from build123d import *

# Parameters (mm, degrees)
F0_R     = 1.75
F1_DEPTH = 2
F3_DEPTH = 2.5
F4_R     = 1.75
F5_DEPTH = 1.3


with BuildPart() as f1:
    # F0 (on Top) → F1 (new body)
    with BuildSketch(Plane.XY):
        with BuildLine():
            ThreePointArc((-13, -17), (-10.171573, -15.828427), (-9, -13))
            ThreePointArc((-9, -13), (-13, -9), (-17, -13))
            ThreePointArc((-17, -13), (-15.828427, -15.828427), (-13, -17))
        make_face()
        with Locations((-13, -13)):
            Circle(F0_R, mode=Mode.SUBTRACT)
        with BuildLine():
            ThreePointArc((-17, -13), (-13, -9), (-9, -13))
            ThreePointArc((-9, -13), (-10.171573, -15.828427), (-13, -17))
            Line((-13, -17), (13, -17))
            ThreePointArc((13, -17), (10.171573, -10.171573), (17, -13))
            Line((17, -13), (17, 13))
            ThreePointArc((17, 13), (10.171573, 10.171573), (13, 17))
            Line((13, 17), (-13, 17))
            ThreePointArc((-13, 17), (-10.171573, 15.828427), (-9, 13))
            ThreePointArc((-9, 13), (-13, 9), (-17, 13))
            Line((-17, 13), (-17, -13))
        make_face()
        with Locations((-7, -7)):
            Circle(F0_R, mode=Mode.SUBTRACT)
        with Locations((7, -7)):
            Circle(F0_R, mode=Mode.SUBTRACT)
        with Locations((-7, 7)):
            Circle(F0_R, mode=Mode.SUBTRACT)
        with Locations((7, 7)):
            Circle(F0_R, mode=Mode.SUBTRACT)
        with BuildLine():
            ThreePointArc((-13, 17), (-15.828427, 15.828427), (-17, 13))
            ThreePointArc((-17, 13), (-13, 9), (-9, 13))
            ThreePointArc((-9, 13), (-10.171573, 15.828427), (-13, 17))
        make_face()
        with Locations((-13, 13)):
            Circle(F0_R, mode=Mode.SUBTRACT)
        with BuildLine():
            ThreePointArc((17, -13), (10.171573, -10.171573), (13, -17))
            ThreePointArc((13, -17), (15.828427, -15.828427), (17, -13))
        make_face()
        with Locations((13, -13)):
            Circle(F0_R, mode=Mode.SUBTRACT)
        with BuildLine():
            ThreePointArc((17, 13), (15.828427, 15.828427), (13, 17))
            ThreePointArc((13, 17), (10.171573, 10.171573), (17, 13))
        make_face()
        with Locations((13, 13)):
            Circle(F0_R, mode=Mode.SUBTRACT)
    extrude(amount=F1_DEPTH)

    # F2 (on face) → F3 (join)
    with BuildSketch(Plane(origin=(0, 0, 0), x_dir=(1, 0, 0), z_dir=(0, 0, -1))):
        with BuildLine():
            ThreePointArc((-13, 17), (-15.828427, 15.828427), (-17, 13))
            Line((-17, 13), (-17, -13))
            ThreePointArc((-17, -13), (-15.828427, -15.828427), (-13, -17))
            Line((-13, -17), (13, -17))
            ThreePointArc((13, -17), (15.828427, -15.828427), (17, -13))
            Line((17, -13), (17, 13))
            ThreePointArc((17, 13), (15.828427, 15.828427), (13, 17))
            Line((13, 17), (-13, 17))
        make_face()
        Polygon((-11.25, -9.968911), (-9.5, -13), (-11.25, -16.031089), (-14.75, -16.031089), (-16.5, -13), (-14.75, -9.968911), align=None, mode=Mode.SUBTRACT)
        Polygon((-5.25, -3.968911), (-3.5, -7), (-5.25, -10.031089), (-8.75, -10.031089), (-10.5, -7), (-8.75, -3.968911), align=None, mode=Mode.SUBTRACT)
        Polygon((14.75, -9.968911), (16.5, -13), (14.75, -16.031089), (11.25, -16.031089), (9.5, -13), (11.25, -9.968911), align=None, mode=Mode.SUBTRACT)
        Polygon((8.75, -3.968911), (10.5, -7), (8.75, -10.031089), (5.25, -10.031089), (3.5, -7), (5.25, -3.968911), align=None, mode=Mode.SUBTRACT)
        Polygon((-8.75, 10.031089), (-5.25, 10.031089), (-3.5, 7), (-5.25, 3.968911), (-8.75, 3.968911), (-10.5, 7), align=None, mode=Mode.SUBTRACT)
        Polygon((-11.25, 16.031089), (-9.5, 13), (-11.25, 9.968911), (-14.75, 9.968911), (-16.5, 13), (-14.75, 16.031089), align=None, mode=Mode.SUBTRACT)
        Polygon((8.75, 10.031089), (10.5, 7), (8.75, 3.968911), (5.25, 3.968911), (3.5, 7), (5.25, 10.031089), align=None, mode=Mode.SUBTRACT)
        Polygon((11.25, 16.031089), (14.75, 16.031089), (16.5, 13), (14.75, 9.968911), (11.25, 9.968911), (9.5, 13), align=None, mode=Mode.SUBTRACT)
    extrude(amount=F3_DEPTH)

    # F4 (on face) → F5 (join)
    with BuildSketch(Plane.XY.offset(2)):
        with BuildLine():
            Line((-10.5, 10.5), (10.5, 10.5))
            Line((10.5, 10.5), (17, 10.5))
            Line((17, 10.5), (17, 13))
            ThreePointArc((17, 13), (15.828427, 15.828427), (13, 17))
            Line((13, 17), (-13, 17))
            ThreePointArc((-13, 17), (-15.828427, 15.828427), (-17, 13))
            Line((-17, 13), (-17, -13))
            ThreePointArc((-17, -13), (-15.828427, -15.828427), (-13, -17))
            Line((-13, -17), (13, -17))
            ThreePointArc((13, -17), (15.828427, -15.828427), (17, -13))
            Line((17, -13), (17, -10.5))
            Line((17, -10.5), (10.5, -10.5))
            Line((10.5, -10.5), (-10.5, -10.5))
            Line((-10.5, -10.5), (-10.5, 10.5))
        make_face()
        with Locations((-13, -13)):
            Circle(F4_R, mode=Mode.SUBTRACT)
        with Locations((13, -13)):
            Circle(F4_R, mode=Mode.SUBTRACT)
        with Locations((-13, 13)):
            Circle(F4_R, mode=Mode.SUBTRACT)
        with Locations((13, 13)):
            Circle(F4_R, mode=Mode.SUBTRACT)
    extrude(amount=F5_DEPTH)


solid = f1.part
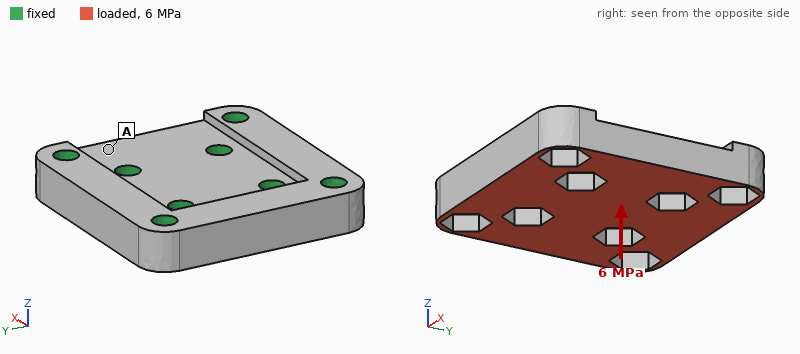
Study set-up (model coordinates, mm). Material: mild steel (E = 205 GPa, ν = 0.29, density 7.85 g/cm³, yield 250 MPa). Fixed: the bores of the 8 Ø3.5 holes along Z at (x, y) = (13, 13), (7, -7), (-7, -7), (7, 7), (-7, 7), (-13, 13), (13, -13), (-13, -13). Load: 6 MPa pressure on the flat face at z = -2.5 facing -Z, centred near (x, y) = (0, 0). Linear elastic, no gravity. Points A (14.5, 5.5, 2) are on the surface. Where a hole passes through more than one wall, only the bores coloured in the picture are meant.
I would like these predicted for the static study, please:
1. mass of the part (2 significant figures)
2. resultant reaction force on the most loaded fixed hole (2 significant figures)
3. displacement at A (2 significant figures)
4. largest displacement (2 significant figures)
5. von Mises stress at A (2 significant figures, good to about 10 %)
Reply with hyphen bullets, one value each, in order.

- 40 g
- 780 N
- 2.4 µm
- 4.3 µm
- 12 MPa
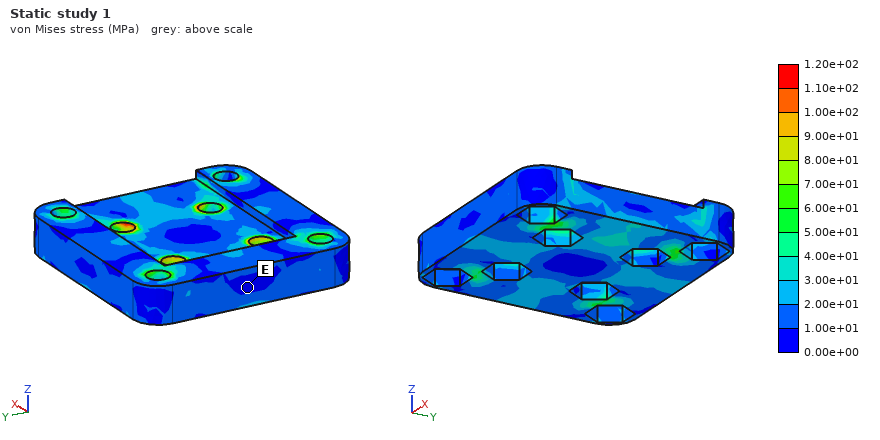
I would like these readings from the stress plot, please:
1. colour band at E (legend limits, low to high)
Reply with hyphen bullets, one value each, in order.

- 0.00e+00 to 1.00e+01 MPa
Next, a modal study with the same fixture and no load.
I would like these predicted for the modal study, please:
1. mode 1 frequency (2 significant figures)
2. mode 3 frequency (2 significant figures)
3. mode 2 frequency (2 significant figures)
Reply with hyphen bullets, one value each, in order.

- 37 kHz
- 39 kHz
- 39 kHz
